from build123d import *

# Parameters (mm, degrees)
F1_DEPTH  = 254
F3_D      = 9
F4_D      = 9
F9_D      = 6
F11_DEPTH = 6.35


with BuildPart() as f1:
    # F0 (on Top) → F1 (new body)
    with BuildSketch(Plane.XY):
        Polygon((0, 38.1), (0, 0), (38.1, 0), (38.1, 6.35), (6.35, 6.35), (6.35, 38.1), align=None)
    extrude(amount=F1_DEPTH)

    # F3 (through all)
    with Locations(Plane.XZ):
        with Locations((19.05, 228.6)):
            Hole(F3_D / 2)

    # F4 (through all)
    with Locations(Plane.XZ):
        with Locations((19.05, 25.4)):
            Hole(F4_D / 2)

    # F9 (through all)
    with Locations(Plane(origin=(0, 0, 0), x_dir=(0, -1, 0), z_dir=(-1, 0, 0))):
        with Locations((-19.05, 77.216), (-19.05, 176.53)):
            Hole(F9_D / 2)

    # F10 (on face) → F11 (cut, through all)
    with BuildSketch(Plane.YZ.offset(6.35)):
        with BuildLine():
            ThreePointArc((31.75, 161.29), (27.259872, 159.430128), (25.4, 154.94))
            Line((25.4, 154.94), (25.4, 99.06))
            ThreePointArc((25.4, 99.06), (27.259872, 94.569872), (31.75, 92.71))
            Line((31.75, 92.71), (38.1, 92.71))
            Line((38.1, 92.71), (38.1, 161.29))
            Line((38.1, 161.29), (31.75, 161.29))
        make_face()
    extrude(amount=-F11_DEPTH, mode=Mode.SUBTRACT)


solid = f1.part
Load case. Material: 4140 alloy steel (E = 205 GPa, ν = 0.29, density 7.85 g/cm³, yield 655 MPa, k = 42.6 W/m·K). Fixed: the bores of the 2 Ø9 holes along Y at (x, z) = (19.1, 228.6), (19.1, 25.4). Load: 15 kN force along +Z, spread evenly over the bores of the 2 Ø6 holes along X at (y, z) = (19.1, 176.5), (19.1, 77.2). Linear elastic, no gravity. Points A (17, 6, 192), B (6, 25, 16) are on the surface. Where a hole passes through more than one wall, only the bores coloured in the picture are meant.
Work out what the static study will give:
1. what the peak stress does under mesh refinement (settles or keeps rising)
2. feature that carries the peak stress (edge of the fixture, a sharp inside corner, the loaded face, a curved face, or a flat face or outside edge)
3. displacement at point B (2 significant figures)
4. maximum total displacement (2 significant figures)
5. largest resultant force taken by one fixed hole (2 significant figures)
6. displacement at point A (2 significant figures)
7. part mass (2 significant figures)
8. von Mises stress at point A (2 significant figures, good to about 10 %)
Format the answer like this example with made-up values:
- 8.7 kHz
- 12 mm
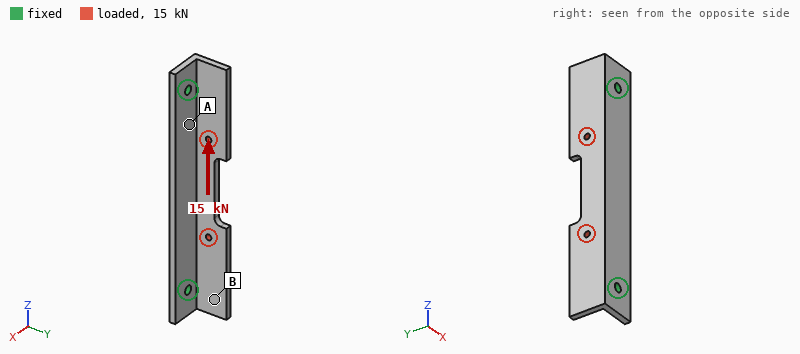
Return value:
- keeps rising
- edge of the fixture
- 16 µm
- 26 µm
- 7.7 kN
- 5.8 µm
- 830 g
- 23 MPa
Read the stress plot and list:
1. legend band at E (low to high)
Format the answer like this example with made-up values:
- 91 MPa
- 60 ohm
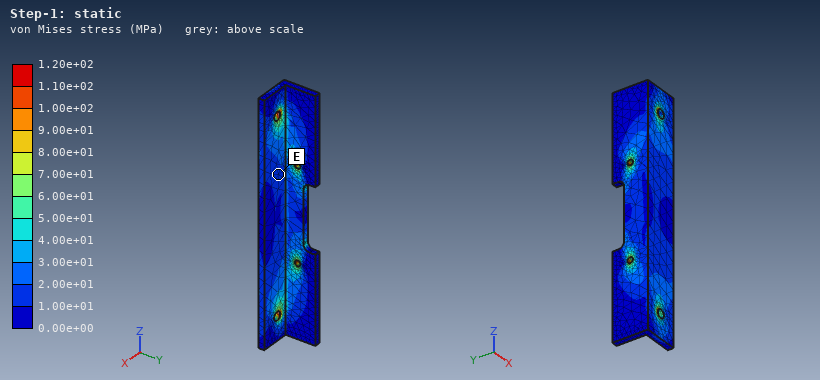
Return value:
- 1.00e+01 to 2.00e+01 MPa
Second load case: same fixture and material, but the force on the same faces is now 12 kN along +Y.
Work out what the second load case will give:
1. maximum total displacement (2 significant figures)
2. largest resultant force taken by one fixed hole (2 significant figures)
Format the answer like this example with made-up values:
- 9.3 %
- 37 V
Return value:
- 0.37 mm
- 9.4 kN
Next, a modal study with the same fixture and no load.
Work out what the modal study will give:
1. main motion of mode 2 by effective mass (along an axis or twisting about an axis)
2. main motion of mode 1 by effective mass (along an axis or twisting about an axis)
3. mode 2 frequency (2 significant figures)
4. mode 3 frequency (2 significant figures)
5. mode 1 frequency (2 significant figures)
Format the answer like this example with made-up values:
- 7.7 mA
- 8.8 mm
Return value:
- along X
- along Y
- 1600 Hz
- 2500 Hz
- 1500 Hz
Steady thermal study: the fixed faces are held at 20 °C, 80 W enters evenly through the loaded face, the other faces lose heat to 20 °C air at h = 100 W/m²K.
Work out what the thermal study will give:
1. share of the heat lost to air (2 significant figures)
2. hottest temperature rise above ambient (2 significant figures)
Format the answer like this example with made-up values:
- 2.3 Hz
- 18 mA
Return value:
- 85 %
- 78 K
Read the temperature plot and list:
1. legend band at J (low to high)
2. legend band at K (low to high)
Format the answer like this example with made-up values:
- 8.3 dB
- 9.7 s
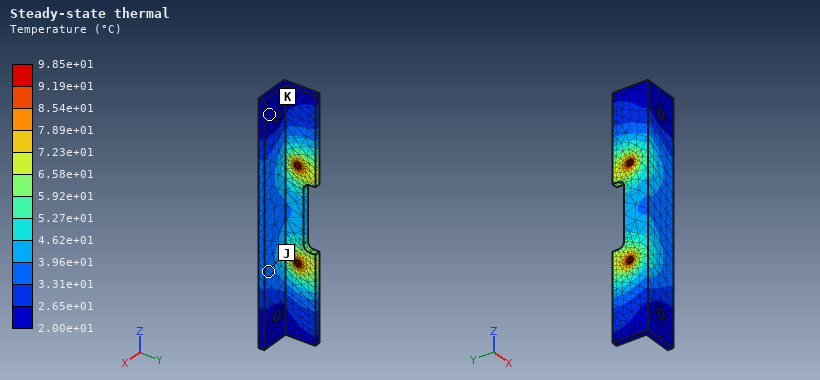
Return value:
- 3.31e+01 to 3.96e+01 °C
- 2.00e+01 to 2.65e+01 °C
